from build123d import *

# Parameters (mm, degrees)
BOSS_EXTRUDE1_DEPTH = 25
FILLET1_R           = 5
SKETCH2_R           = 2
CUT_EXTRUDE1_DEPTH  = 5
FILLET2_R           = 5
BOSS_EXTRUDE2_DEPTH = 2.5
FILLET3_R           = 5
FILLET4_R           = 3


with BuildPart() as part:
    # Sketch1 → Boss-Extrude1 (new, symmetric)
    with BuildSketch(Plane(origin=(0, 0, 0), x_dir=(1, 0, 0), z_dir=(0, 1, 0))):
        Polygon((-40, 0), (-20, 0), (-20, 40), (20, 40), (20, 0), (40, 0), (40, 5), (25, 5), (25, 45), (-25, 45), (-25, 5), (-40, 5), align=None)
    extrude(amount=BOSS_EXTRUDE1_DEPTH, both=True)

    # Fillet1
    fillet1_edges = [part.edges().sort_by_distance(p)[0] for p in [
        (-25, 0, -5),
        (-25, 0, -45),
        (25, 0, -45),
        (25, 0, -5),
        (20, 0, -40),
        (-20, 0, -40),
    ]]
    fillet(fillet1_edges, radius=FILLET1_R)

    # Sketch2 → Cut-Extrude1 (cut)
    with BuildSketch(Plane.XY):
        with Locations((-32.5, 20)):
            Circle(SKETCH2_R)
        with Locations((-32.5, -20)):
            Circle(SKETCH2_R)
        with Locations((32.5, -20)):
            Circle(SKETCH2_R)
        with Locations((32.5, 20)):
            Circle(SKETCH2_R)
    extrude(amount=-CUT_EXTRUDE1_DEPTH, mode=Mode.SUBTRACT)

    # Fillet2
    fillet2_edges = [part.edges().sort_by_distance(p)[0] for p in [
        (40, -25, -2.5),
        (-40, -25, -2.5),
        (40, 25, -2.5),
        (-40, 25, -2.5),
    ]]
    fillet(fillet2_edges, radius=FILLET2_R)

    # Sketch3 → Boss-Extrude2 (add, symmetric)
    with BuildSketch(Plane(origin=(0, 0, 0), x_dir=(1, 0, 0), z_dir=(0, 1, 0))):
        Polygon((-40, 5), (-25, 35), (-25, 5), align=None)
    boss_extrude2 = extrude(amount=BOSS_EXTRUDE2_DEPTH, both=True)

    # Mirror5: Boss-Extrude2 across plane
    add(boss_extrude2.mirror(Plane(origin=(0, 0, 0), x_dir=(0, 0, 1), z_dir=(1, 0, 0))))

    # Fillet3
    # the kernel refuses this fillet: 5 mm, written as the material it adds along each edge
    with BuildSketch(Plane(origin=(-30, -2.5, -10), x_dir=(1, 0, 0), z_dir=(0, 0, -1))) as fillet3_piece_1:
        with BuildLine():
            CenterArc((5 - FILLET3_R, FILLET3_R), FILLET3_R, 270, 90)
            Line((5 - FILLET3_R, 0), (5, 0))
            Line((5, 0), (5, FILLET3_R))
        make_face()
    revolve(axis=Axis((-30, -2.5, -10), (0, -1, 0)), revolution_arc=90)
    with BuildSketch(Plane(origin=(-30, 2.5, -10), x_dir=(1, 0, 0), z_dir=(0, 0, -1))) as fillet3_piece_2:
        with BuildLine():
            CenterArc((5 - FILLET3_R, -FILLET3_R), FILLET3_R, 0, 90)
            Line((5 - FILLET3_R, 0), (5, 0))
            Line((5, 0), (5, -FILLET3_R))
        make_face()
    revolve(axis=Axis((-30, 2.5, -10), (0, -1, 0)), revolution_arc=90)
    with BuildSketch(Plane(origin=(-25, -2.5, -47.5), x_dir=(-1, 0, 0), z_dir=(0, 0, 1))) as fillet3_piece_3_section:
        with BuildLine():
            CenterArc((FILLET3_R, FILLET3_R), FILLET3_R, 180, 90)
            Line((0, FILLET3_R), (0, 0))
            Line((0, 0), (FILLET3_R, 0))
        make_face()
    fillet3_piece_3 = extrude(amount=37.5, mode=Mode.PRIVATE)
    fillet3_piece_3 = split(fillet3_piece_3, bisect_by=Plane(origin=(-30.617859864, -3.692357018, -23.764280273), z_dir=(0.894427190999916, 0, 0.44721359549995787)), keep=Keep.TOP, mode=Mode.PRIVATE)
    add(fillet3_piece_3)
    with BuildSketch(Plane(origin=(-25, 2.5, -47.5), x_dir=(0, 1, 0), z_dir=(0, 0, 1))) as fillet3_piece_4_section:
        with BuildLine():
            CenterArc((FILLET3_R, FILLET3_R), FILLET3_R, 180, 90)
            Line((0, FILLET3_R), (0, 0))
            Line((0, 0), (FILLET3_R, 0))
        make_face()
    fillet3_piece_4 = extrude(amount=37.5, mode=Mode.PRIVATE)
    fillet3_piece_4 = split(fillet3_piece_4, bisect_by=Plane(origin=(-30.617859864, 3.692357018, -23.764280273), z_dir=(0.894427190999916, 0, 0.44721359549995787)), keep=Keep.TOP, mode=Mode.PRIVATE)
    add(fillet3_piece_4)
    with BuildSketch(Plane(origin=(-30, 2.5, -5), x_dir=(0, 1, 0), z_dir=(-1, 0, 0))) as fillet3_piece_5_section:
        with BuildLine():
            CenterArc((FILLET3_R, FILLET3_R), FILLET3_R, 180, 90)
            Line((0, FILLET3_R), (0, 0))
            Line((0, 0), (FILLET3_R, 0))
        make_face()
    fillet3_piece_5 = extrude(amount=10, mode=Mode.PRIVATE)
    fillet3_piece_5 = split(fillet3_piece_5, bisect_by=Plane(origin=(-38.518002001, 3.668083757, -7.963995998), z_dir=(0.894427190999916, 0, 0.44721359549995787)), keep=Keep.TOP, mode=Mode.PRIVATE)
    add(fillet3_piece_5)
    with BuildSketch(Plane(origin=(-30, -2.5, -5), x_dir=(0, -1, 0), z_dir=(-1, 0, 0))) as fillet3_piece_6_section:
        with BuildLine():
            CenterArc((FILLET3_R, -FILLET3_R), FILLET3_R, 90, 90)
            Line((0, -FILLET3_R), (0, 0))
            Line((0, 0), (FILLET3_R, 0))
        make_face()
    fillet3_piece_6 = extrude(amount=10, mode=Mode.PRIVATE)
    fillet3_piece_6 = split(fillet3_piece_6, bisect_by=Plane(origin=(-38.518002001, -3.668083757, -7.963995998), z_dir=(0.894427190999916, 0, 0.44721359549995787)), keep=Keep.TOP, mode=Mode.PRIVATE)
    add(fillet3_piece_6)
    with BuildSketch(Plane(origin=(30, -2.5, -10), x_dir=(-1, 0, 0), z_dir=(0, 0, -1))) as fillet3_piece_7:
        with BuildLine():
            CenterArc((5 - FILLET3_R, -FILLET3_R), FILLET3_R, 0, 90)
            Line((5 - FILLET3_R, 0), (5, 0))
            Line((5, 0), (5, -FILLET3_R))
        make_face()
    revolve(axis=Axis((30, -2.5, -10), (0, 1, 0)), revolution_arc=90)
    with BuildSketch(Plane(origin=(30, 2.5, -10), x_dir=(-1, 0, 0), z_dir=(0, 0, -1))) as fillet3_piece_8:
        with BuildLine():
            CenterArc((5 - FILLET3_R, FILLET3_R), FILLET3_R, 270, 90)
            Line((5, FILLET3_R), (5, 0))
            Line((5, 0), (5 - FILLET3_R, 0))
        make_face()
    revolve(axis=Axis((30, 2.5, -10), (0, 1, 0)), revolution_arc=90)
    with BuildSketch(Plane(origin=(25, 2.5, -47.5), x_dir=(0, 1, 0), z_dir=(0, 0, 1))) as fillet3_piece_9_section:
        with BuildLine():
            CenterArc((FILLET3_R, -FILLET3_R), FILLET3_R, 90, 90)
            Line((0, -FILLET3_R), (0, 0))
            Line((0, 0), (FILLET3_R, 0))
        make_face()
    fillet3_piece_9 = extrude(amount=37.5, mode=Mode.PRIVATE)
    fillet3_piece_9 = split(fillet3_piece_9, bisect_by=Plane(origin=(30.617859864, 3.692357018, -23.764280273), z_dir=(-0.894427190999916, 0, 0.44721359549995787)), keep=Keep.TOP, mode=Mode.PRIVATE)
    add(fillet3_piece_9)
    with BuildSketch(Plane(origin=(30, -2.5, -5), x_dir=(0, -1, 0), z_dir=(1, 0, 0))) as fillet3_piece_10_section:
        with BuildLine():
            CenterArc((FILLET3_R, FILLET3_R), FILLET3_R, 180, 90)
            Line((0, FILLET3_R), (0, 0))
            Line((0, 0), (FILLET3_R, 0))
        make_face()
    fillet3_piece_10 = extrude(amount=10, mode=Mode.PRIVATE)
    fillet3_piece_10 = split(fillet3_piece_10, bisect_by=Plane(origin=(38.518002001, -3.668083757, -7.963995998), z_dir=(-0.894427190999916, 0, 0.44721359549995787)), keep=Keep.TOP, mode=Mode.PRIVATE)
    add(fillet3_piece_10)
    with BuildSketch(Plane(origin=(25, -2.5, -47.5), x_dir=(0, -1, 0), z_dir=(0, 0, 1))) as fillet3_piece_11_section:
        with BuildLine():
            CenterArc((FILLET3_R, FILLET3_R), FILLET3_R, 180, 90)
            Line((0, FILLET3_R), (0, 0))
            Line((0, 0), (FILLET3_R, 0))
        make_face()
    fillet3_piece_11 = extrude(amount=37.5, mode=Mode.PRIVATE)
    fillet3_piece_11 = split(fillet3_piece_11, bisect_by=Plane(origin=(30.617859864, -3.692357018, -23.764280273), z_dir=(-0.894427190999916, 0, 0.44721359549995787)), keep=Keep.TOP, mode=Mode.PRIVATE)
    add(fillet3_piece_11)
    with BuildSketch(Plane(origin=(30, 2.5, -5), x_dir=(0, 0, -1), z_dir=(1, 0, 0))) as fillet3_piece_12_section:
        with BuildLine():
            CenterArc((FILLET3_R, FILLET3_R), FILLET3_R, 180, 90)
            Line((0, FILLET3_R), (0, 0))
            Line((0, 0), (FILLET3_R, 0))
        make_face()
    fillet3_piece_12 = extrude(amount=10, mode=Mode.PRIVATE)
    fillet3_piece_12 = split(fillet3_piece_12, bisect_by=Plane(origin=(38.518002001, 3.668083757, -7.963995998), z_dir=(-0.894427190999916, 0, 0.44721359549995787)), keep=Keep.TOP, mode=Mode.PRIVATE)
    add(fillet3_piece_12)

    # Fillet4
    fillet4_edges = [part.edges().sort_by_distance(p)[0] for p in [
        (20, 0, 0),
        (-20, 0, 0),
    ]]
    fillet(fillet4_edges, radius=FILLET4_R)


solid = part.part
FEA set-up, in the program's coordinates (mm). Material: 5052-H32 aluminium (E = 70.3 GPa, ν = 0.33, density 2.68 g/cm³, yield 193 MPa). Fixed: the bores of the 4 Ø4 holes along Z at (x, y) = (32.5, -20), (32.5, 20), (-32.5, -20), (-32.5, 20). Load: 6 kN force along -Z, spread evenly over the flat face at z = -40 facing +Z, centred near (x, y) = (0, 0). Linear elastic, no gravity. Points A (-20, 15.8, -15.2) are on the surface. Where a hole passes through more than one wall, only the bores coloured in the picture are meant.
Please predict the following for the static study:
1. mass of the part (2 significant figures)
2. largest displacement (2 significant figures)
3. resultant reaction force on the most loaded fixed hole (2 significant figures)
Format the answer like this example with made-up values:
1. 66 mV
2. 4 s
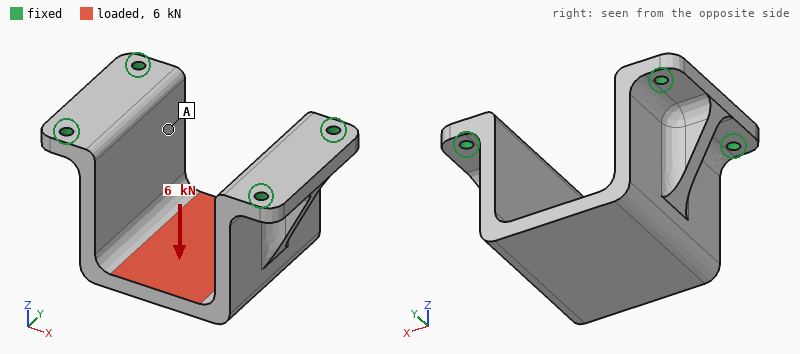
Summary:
1. 120 g
2. 0.10 mm
3. 1.7 kN
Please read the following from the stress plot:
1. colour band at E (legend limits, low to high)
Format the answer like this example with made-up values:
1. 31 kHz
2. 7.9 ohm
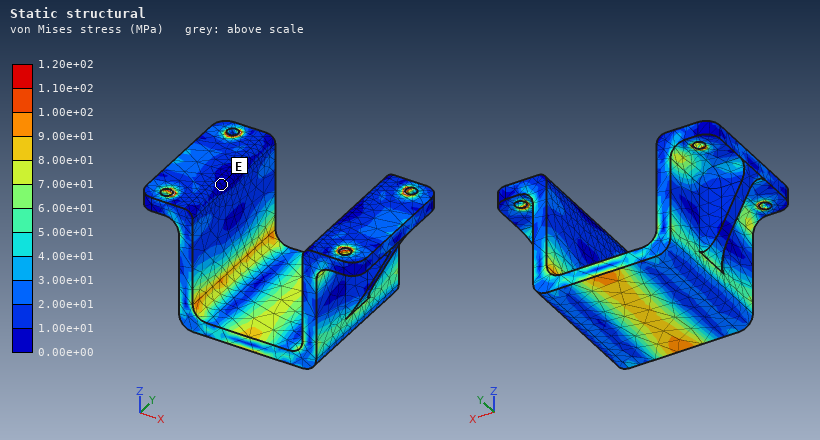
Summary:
1. 0.00e+00 to 1.00e+01 MPa
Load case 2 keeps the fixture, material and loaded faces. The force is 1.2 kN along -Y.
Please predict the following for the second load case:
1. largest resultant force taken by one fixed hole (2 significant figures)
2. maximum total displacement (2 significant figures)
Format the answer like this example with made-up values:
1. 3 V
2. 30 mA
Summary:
1. 660 N
2. 25 µm
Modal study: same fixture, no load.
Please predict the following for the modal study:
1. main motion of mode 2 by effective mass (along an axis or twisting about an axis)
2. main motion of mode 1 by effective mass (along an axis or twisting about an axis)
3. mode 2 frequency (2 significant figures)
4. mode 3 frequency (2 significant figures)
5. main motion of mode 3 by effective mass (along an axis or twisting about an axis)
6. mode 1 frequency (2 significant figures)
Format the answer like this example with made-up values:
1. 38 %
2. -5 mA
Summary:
1. along Y
2. along X
3. 4900 Hz
4. 5200 Hz
5. twisting about Z
6. 2500 Hz
